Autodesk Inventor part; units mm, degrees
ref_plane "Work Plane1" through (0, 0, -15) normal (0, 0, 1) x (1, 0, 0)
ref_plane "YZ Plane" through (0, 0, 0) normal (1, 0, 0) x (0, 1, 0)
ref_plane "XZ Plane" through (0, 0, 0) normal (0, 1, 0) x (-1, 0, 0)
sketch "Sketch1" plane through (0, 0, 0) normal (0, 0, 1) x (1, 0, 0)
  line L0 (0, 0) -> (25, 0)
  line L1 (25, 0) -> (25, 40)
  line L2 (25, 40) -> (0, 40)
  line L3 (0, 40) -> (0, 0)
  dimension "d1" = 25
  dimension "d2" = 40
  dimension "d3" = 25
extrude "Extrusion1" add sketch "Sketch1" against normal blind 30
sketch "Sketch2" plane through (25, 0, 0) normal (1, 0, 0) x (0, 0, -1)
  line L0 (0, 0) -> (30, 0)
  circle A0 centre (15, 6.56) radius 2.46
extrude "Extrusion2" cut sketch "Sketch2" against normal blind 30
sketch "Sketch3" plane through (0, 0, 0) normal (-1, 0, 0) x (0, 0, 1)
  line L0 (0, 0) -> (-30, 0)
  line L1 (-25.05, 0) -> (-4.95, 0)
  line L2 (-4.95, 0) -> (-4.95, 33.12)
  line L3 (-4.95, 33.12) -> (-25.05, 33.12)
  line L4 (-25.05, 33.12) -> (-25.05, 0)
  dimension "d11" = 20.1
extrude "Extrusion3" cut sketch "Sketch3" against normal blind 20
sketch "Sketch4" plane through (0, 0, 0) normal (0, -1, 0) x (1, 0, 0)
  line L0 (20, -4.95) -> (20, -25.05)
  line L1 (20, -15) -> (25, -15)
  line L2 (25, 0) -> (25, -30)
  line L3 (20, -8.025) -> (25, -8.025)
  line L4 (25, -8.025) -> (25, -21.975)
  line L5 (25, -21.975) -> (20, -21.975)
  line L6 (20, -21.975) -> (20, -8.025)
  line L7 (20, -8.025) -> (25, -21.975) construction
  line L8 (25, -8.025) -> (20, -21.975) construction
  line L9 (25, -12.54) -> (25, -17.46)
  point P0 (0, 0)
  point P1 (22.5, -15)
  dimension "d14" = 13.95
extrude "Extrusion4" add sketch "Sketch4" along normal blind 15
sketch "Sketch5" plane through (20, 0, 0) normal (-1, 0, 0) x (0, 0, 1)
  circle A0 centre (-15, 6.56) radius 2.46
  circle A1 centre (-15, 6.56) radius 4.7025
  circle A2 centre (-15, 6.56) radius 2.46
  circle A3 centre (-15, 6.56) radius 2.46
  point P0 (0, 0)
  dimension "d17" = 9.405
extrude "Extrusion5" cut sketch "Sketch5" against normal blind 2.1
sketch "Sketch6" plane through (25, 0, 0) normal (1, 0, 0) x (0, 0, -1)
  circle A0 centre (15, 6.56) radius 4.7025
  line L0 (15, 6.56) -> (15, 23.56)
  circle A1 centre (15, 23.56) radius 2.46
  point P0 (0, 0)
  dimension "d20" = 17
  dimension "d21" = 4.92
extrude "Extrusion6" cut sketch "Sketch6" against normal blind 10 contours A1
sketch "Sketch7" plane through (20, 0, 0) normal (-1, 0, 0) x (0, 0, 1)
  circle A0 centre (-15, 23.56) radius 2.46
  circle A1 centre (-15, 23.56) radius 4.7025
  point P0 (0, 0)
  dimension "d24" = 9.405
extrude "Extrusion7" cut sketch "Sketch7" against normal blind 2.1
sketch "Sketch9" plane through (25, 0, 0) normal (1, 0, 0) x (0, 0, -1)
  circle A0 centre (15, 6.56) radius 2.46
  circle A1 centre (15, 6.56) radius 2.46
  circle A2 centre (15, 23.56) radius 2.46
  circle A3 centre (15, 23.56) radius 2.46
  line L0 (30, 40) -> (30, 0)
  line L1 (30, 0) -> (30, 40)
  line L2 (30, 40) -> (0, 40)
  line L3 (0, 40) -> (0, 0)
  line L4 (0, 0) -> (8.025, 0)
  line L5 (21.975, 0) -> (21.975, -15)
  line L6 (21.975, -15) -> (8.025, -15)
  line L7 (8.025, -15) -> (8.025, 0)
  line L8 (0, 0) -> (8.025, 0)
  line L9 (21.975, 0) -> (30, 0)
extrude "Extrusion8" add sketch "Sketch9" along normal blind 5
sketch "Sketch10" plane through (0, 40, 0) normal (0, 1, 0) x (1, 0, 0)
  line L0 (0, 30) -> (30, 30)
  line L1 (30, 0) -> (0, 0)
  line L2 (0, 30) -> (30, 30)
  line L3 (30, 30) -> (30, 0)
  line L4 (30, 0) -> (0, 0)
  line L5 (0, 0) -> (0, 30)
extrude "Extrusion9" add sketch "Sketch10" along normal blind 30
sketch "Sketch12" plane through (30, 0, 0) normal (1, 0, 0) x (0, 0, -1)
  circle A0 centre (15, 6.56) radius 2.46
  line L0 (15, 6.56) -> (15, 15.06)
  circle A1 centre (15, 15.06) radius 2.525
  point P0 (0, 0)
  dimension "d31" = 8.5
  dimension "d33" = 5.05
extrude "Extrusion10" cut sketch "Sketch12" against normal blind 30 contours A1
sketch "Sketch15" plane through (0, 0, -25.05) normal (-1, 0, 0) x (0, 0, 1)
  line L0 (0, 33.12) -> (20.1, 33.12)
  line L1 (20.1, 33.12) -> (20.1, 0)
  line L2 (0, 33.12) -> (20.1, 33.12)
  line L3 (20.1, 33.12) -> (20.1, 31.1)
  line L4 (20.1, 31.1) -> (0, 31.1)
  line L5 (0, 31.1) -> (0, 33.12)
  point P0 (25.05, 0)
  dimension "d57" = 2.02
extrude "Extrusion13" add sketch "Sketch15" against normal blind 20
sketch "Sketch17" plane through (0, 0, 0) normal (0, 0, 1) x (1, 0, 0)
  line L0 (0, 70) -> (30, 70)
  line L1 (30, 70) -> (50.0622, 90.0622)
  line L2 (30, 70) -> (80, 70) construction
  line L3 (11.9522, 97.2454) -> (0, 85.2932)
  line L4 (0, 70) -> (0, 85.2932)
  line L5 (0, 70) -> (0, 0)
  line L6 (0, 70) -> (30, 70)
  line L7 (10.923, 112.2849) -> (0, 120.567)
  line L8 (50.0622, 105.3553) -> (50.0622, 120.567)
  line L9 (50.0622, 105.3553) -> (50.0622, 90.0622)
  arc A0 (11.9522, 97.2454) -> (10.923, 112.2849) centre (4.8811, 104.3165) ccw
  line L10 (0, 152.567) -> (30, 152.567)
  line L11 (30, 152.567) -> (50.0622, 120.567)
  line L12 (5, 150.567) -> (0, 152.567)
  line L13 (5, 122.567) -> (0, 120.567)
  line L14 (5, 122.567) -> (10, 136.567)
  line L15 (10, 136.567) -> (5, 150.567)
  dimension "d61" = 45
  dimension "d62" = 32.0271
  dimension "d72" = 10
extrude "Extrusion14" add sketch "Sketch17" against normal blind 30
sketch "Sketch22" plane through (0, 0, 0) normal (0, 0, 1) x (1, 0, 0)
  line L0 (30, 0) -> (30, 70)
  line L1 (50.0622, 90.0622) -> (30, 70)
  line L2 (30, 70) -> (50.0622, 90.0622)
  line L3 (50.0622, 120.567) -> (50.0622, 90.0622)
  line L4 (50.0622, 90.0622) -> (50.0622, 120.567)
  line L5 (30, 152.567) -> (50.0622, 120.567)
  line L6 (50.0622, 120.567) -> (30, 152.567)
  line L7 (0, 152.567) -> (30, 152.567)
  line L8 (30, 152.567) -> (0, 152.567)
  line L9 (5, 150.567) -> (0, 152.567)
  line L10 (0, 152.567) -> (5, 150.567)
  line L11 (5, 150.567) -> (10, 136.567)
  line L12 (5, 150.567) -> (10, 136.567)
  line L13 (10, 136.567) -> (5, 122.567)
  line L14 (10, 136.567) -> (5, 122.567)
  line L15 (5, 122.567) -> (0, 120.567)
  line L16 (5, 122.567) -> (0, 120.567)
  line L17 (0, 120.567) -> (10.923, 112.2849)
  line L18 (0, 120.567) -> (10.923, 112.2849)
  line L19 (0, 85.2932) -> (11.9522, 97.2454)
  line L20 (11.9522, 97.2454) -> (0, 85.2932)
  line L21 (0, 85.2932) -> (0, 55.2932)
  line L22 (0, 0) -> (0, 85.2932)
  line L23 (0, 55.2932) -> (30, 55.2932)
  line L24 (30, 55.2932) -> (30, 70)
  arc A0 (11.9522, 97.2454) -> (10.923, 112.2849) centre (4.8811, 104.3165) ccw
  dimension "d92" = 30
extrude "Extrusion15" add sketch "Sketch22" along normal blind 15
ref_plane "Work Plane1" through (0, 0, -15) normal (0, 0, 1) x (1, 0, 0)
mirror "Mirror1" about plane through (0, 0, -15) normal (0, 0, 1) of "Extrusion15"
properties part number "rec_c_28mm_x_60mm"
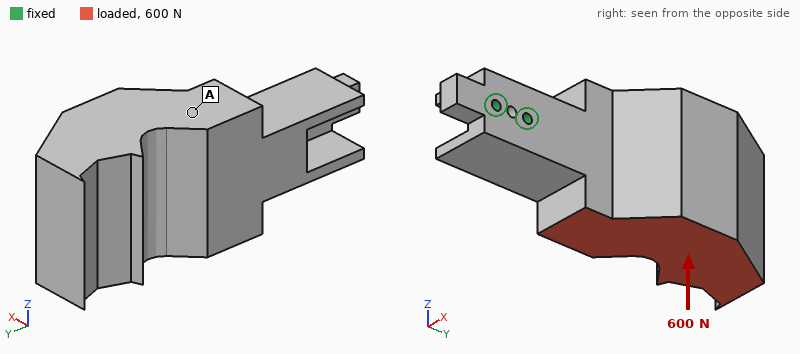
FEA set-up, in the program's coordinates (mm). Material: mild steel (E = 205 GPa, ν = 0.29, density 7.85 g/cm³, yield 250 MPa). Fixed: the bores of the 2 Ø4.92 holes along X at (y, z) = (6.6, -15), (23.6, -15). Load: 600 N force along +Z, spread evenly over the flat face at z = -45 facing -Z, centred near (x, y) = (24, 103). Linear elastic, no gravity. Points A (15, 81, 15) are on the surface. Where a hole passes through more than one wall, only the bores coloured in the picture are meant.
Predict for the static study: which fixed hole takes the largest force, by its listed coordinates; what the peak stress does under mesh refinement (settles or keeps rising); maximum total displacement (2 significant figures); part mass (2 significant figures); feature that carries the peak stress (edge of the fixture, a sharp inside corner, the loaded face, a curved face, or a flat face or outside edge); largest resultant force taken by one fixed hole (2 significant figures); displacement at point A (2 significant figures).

(23.6, -15)
keeps rising
43 µm
2.0 kg
edge of the fixture
2.7 kN
20 µm
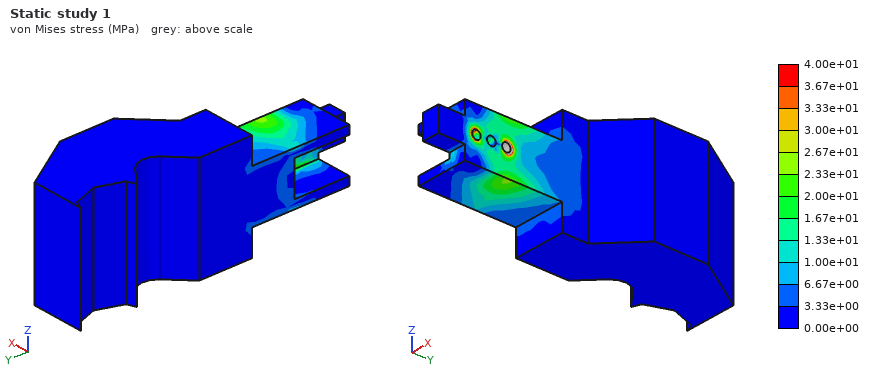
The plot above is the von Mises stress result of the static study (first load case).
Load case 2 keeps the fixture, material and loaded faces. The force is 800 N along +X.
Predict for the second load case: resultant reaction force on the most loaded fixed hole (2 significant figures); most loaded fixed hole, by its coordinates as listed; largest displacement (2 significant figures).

3.3 kN
(23.6, -15)
91 µm
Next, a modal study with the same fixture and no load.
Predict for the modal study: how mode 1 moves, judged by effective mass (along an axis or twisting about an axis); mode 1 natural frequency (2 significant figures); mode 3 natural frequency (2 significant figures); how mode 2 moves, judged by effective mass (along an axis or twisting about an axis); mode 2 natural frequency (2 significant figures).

along X
480 Hz
1300 Hz
along Z
550 Hz
